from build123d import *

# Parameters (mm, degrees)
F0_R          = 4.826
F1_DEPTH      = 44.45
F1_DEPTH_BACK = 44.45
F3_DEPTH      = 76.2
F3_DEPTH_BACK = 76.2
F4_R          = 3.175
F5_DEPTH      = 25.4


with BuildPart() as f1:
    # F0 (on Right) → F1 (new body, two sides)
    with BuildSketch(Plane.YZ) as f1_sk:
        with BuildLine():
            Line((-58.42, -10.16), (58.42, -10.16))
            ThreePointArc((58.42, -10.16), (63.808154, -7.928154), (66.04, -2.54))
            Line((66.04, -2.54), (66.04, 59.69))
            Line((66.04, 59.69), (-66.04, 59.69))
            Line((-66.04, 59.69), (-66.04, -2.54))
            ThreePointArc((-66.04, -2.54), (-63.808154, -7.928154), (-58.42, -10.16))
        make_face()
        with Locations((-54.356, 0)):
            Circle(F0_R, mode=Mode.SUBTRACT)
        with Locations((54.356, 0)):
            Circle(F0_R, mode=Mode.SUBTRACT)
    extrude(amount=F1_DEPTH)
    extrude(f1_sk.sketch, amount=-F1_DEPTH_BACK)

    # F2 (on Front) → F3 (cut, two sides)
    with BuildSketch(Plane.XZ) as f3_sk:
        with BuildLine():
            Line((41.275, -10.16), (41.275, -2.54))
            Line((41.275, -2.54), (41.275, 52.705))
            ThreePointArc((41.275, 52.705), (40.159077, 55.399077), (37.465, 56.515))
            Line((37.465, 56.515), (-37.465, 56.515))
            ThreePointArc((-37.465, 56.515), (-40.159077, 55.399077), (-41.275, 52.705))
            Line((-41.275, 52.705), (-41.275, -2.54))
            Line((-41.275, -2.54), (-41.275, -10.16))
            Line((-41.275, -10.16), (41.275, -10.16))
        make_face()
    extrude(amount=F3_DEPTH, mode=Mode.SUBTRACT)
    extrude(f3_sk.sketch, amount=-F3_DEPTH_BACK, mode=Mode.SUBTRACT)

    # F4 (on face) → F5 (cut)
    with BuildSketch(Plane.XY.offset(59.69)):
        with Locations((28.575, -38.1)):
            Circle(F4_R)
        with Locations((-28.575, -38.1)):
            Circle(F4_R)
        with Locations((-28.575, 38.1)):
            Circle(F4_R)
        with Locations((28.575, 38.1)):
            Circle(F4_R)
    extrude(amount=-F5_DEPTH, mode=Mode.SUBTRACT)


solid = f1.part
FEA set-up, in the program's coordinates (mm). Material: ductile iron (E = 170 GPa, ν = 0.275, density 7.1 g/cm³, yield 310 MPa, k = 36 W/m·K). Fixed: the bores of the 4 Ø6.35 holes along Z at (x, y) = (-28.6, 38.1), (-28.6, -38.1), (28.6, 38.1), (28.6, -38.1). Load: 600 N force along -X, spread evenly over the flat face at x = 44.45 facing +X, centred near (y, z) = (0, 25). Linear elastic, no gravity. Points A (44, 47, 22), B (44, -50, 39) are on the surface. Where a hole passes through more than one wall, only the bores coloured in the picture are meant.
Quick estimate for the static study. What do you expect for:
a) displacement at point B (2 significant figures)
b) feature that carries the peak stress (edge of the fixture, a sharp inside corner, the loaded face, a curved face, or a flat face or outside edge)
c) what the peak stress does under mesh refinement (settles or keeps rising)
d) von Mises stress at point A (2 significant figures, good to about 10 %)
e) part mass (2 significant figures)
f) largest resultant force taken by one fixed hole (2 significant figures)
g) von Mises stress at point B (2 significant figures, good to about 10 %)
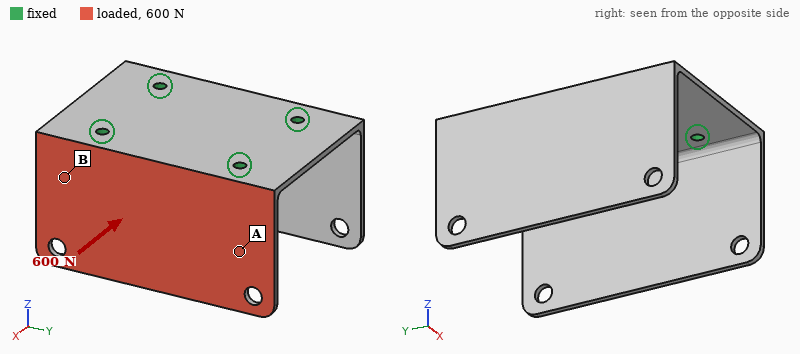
0.13 mm
edge of the fixture
keeps rising
18 MPa
660 g
220 N
41 MPa
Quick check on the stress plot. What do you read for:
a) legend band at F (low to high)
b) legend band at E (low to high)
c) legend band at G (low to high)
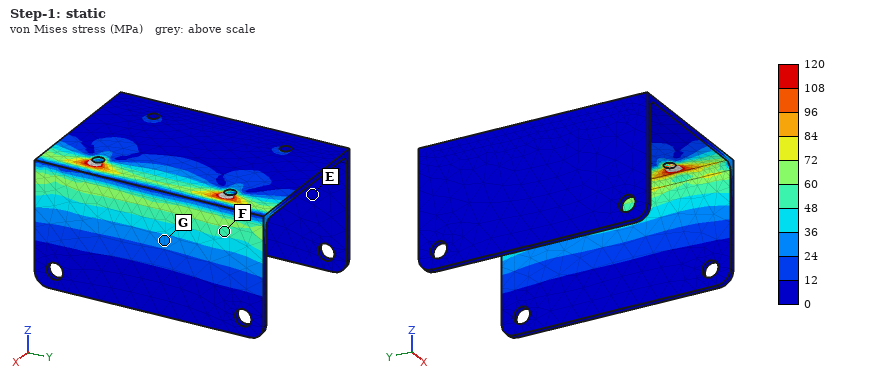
48 to 60 MPa
0 to 12 MPa
24 to 36 MPa
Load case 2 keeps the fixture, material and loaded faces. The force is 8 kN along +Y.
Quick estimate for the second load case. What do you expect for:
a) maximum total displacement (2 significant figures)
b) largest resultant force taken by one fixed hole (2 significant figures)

0.38 mm
5.3 kN
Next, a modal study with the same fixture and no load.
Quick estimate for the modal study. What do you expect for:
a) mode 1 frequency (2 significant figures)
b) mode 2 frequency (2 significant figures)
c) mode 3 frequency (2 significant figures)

430 Hz
440 Hz
770 Hz
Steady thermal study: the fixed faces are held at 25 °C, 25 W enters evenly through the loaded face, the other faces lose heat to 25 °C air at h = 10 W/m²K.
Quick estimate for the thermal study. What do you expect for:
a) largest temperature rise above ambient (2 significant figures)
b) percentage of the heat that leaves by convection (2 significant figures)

68 K
30 %
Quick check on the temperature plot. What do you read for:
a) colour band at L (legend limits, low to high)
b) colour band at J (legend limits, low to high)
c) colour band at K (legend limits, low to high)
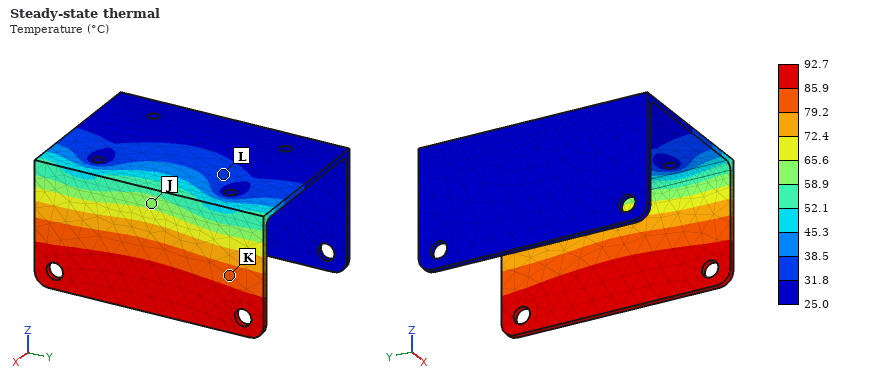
31.8 to 38.5 °C
58.9 to 65.6 °C
79.2 to 85.9 °C
